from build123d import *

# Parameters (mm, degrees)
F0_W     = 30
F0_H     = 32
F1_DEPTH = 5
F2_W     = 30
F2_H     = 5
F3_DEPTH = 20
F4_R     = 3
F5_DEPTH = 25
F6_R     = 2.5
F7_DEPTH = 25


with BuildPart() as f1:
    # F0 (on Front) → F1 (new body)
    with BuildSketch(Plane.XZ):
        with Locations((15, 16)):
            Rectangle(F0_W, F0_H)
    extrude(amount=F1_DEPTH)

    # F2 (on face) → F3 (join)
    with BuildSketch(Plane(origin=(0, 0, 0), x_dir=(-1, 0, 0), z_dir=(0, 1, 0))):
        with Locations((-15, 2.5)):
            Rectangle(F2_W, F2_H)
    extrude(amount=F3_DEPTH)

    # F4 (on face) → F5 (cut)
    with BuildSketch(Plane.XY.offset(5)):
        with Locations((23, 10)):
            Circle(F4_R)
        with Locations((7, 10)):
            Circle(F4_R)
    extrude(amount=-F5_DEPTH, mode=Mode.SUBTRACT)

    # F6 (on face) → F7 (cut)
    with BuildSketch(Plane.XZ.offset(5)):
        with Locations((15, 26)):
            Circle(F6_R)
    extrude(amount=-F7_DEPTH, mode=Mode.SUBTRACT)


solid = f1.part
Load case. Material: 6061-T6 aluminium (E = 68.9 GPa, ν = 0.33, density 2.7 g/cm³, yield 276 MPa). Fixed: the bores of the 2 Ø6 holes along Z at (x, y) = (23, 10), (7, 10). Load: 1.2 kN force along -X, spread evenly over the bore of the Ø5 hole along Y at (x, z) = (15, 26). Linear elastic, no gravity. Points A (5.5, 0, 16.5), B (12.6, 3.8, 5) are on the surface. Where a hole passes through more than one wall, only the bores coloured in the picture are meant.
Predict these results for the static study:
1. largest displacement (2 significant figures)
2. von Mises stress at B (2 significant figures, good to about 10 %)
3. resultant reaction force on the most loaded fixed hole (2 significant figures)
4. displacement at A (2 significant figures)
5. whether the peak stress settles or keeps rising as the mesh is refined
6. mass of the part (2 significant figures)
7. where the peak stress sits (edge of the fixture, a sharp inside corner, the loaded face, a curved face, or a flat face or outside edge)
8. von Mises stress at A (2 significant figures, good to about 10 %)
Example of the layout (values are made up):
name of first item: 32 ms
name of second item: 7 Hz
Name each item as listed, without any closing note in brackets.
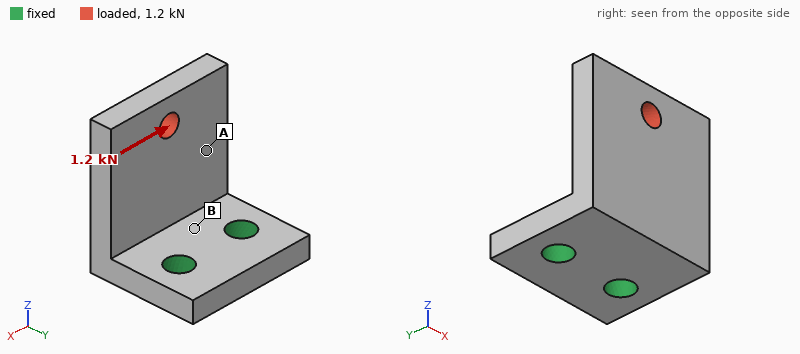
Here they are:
largest displacement: 0.14 mm
von Mises stress at B: 83 MPa
resultant reaction force on the most loaded fixed hole: 1.6 kN
displacement at A: 0.069 mm
whether the peak stress settles or keeps rising as the mesh is refined: keeps rising
mass of the part: 20 g
where the peak stress sits: edge of the fixture
von Mises stress at A: 31 MPa
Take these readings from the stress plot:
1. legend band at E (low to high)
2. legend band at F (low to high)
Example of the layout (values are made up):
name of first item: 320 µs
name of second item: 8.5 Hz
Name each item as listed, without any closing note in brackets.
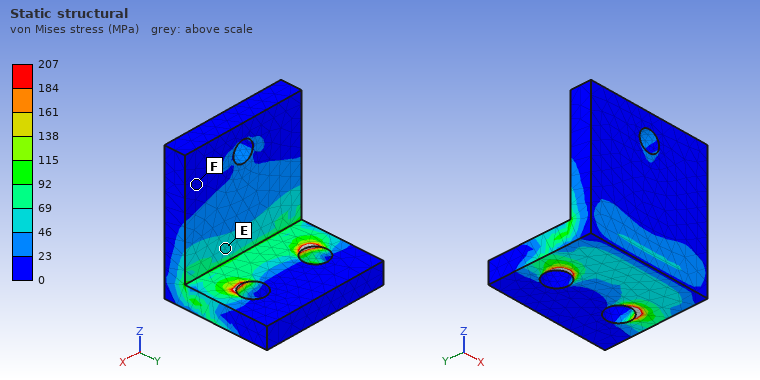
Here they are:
legend band at E: 46 to 69 MPa
legend band at F: 0 to 23 MPa
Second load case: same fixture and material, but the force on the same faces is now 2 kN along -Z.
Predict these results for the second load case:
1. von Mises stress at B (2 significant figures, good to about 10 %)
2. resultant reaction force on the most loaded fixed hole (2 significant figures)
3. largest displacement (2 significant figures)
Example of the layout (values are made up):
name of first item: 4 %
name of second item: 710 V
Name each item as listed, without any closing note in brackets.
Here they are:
von Mises stress at B: 78 MPa
resultant reaction force on the most loaded fixed hole: 1.0 kN
largest displacement: 0.17 mm
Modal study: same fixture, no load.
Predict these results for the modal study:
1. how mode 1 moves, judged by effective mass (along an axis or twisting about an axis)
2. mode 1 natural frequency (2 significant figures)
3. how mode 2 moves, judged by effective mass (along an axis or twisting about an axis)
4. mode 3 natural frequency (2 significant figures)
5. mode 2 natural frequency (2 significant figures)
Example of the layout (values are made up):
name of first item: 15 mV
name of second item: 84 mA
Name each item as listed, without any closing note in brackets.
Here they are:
how mode 1 moves, judged by effective mass: along Y
mode 1 natural frequency: 3200 Hz
how mode 2 moves, judged by effective mass: along X
mode 3 natural frequency: 10000 Hz
mode 2 natural frequency: 6400 Hz
